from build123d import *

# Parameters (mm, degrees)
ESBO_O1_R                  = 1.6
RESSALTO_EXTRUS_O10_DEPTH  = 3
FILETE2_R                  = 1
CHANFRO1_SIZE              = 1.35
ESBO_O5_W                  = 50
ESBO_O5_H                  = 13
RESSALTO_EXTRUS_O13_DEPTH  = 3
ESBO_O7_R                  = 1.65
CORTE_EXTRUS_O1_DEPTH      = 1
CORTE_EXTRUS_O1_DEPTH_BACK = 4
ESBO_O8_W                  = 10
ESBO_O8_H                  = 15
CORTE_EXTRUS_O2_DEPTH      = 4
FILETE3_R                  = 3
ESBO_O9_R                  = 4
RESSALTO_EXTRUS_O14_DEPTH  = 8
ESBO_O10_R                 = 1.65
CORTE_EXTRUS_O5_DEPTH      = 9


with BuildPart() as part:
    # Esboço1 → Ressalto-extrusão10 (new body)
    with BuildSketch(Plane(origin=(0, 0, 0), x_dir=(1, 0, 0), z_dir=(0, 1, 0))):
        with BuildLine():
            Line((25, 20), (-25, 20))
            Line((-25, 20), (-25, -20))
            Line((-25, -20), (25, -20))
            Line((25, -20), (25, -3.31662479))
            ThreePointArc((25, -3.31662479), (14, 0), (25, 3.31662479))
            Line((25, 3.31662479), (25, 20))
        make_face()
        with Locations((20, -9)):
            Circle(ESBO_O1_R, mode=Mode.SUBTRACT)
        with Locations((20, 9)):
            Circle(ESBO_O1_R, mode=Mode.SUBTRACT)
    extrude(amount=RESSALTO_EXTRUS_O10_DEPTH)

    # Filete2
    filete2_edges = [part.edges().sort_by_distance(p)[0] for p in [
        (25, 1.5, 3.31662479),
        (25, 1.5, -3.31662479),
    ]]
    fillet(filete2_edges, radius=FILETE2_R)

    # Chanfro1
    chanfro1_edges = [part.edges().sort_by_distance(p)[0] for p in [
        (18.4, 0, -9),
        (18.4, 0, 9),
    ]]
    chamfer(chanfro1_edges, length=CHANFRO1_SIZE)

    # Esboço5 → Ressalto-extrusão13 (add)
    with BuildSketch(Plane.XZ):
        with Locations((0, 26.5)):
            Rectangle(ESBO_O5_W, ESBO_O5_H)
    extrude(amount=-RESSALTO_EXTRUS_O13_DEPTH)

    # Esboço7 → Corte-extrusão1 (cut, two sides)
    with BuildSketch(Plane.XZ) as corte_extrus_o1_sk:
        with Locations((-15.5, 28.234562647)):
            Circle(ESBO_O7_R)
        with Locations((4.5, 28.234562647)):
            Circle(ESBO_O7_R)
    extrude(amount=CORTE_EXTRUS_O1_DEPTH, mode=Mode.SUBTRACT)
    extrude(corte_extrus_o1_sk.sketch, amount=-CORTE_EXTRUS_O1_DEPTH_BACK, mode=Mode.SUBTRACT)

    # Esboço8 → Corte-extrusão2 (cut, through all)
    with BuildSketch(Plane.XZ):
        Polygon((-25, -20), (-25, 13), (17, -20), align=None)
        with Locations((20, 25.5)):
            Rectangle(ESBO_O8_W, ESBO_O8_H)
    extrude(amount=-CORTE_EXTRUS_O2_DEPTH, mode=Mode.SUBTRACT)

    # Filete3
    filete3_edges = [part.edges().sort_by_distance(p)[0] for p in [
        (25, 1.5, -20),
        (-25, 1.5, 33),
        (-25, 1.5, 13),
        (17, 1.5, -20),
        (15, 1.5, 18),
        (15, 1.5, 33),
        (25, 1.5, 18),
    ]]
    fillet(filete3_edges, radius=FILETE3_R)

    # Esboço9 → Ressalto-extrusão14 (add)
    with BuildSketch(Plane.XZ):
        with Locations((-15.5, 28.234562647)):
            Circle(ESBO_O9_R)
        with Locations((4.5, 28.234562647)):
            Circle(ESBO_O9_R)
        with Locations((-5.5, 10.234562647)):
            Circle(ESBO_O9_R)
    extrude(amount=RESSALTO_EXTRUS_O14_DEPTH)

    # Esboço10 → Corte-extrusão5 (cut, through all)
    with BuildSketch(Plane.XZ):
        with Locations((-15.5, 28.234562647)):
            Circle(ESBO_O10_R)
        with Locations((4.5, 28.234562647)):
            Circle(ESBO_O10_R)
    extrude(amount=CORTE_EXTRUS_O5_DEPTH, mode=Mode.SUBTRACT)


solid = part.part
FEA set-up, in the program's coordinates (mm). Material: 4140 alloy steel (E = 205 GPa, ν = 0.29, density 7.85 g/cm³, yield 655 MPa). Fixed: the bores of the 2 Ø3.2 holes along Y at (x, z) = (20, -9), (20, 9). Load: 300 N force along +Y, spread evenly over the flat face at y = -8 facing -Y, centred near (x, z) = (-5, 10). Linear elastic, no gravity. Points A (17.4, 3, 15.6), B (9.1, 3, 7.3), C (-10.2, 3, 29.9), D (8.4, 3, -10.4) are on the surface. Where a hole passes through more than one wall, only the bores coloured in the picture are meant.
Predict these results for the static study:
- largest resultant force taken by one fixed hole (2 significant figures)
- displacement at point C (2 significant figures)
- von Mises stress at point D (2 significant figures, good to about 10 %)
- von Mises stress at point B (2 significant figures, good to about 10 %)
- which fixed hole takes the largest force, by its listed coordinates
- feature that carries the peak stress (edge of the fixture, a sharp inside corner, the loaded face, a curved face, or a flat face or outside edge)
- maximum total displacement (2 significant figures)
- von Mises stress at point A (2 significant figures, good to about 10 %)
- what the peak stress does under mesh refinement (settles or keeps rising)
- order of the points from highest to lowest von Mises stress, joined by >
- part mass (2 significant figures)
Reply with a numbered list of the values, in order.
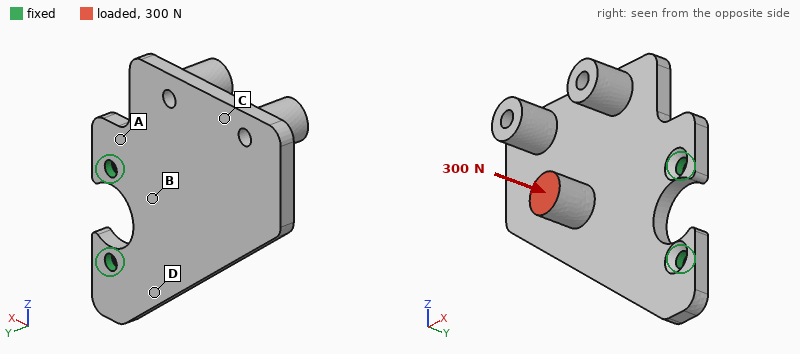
1. 270 N
2. 0.27 mm
3. 110 MPa
4. 77 MPa
5. (20, 9)
6. edge of the fixture
7. 0.42 mm
8. 180 MPa
9. keeps rising
10. A > D > B > C
11. 47 g
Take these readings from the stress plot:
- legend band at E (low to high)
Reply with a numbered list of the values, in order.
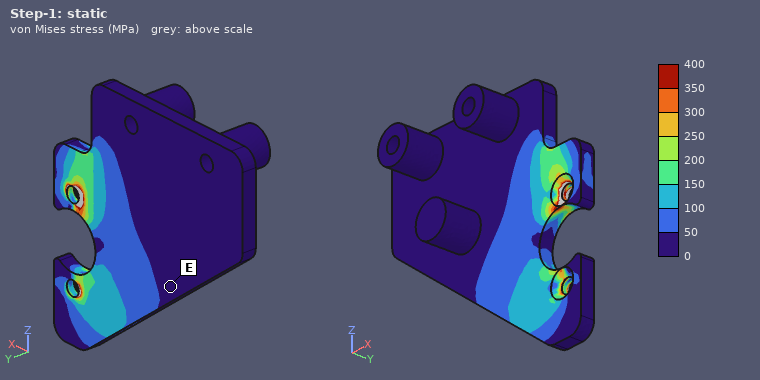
1. 0 to 50 MPa
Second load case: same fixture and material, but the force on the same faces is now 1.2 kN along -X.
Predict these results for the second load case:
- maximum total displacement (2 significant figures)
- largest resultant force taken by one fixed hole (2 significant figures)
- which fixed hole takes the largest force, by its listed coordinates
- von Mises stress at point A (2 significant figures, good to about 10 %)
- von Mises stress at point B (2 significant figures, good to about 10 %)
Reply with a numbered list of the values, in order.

1. 0.85 mm
2. 1.2 kN
3. (20, 9)
4. 300 MPa
5. 160 MPa
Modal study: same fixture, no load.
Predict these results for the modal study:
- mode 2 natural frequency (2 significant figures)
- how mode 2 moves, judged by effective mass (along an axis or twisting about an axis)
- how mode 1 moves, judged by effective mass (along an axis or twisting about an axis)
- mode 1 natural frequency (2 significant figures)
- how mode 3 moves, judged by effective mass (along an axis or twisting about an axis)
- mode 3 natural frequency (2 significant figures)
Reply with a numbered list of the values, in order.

1. 2700 Hz
2. twisting about X
3. along Y
4. 850 Hz
5. along Y
6. 4900 Hz
